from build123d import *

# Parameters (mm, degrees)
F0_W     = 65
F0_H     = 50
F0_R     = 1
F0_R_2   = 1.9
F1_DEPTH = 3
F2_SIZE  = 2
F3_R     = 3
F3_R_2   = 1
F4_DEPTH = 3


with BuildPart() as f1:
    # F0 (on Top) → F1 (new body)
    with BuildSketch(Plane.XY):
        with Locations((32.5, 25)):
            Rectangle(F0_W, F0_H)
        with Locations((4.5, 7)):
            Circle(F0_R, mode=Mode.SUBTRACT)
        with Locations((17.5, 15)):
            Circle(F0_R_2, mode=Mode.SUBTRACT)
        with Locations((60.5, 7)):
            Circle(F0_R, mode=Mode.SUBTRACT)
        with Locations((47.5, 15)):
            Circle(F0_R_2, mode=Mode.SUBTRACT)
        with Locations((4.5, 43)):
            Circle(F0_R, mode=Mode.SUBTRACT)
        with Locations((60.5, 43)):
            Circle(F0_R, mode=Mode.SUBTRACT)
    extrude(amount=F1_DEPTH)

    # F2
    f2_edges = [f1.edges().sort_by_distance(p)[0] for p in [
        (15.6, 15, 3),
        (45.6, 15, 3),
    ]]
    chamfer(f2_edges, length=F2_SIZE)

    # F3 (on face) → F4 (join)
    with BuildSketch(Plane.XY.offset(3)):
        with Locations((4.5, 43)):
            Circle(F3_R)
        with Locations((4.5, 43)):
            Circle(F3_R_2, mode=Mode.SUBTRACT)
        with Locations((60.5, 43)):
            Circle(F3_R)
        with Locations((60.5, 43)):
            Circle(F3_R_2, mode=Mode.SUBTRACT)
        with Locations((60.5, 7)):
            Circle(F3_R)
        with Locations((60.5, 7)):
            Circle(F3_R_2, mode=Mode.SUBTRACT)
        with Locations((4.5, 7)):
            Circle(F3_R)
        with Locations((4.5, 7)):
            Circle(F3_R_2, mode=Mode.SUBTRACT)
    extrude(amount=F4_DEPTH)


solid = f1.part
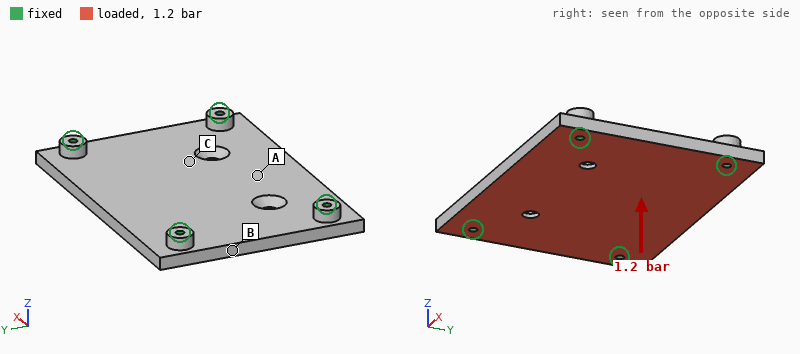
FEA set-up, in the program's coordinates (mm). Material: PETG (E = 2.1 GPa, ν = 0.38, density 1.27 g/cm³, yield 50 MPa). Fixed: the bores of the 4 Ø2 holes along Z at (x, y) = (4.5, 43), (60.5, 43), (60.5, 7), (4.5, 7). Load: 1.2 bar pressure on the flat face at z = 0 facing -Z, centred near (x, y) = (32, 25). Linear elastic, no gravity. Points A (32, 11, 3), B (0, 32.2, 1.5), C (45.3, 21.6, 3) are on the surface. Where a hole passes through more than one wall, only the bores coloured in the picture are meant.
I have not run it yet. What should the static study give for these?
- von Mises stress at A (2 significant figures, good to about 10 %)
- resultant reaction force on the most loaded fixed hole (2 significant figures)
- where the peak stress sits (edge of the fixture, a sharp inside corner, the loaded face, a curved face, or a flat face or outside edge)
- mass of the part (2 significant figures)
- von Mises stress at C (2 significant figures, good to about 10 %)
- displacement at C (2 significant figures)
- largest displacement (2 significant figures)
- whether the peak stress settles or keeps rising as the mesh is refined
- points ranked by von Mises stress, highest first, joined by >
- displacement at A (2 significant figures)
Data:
10.0 MPa
100 N
edge of the fixture
13 g
5.9 MPa
0.62 mm
0.83 mm
keeps rising
A > C > B
0.78 mm
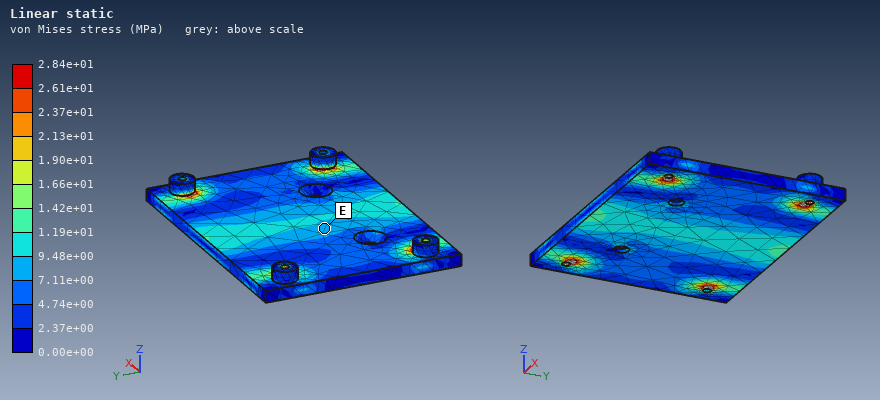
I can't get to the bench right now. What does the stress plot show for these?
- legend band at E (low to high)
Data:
7.11e+00 to 9.48e+00 MPa
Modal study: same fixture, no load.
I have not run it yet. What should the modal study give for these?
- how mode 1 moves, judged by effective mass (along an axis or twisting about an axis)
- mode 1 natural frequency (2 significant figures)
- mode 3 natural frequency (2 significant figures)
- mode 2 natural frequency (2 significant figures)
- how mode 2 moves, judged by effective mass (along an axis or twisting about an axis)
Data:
along Z
1100 Hz
2400 Hz
1600 Hz
twisting about X
